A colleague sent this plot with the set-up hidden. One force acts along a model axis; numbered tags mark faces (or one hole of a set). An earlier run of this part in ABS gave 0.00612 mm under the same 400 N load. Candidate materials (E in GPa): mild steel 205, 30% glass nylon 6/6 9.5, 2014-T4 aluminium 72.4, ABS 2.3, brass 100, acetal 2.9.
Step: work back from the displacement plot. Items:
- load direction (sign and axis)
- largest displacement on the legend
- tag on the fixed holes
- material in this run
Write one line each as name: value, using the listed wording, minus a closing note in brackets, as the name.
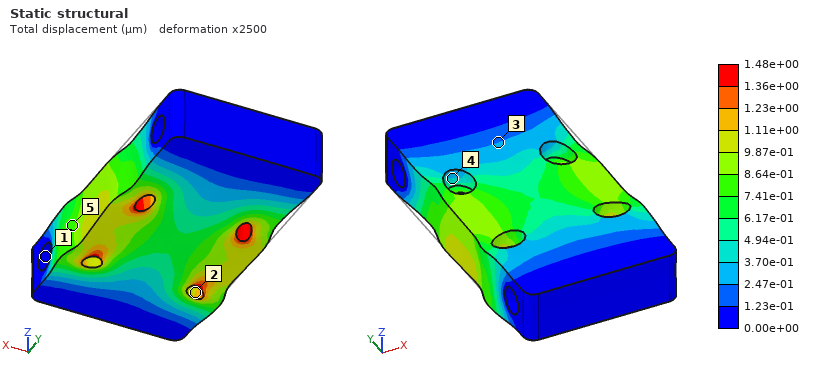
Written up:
load direction: -Y
largest displacement on the legend: 1.48e+00 µm
tag on the fixed holes: 1
material in this run: 30% glass nylon 6/6
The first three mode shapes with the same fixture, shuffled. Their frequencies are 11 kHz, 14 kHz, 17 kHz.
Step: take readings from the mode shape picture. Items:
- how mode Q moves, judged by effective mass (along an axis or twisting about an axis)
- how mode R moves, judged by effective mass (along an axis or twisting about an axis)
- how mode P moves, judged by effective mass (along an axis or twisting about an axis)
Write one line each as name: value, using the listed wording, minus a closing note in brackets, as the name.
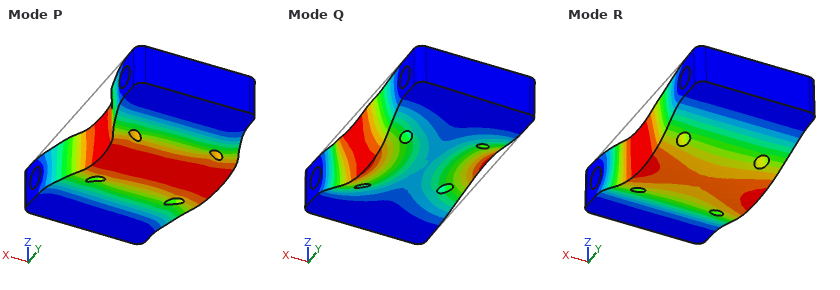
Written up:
how mode Q moves, judged by effective mass: twisting about Y
how mode R moves, judged by effective mass: along Z
how mode P moves, judged by effective mass: along X
